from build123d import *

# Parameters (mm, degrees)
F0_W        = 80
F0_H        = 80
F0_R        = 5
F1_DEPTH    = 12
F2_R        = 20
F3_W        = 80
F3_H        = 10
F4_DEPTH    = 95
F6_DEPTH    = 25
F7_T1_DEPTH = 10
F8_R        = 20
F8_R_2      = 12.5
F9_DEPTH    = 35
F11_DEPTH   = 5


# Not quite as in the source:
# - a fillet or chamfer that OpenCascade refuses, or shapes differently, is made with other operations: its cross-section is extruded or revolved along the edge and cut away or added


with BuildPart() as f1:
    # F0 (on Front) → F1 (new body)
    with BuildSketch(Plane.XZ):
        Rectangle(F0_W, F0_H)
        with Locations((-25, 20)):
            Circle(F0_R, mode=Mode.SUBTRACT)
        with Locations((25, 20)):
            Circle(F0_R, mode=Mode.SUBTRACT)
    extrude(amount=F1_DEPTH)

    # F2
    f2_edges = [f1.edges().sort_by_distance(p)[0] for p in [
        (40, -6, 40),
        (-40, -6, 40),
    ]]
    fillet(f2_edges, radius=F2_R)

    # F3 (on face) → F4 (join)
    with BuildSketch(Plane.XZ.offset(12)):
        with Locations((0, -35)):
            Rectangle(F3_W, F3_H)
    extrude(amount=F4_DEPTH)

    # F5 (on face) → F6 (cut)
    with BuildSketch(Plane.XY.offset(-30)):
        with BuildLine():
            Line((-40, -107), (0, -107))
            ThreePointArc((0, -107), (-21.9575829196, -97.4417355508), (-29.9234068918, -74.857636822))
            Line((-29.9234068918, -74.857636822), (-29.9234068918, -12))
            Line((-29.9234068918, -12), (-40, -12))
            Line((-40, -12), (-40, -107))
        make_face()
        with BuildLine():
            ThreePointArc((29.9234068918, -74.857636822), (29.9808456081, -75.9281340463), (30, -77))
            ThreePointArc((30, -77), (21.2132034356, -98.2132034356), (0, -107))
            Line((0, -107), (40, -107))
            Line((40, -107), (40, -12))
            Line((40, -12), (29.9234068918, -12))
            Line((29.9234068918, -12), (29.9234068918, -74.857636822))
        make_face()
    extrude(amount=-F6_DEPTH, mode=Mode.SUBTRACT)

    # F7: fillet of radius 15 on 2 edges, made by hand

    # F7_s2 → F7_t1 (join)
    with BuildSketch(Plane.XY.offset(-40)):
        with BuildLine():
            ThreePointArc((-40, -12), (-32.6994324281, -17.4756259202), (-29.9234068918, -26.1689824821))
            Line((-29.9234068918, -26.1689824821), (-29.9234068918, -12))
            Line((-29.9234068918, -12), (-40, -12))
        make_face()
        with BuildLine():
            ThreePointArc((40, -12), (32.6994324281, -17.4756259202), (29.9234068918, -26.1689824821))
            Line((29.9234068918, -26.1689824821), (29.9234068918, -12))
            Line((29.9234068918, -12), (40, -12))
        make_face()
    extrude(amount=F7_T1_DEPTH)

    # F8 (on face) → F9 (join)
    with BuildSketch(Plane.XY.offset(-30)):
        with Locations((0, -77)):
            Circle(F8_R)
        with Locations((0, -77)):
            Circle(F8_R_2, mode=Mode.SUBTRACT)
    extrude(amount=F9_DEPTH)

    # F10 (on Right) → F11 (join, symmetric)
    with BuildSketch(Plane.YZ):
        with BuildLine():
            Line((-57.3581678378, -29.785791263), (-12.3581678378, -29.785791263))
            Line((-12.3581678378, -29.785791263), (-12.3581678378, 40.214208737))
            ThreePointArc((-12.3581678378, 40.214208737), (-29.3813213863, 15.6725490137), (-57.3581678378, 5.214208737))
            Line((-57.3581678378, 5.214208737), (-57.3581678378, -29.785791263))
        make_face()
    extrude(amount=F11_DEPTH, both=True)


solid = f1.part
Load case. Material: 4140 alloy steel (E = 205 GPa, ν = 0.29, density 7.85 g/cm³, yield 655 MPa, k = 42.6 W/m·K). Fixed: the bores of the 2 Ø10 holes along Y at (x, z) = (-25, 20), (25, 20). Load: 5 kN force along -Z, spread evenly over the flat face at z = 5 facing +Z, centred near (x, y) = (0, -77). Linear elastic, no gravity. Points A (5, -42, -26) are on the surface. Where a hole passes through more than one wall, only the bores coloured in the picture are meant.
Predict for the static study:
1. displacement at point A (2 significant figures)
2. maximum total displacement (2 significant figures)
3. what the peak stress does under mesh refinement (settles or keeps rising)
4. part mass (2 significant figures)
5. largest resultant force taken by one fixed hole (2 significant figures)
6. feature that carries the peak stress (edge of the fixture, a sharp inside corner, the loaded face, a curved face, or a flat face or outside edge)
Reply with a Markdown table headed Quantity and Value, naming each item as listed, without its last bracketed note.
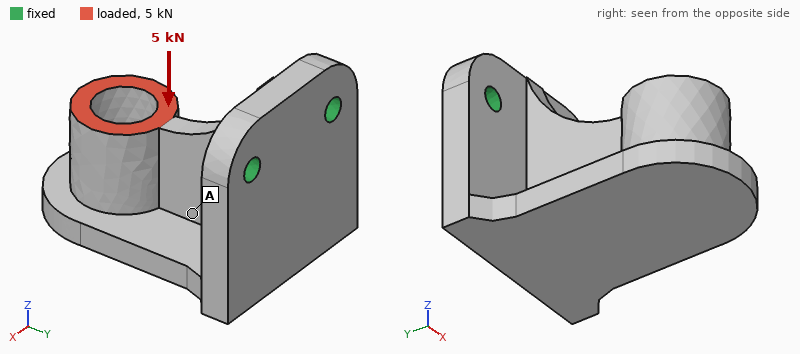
| Quantity | Value |
|---|---|
| displacement at point A | 0.41 mm |
| maximum total displacement | 1.6 mm |
| what the peak stress does under mesh refinement | keeps rising |
| part mass | 1.4 kg |
| largest resultant force taken by one fixed hole | 2.6 kN |
| feature that carries the peak stress | edge of the fixture |
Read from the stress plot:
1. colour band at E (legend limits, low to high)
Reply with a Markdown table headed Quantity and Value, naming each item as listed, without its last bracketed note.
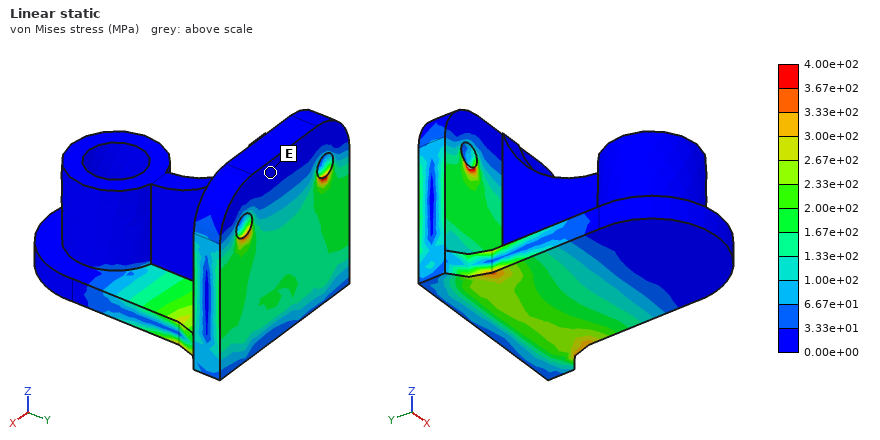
| Quantity | Value |
|---|---|
| colour band at E | 0.00e+00 to 3.33e+01 MPa |
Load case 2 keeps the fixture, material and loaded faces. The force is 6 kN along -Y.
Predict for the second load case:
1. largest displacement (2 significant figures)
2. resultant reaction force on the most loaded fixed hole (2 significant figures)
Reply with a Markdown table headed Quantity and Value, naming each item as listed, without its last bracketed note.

| Quantity | Value |
|---|---|
| largest displacement | 1.1 mm |
| resultant reaction force on the most loaded fixed hole | 3.0 kN |
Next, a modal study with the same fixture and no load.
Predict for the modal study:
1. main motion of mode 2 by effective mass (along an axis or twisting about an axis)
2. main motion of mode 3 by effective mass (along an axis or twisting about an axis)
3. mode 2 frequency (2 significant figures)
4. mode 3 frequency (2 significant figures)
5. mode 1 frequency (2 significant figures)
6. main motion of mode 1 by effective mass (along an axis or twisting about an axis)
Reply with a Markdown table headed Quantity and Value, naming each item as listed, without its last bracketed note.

| Quantity | Value |
|---|---|
| main motion of mode 2 by effective mass | along X |
| main motion of mode 3 by effective mass | along Y |
| mode 2 frequency | 840 Hz |
| mode 3 frequency | 1100 Hz |
| mode 1 frequency | 470 Hz |
| main motion of mode 1 by effective mass | along Z |
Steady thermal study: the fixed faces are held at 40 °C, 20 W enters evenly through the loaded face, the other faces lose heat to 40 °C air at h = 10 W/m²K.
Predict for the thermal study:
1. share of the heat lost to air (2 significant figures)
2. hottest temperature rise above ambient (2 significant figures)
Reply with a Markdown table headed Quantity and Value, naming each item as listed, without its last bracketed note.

| Quantity | Value |
|---|---|
| share of the heat lost to air | 52 % |
| hottest temperature rise above ambient | 59 K |
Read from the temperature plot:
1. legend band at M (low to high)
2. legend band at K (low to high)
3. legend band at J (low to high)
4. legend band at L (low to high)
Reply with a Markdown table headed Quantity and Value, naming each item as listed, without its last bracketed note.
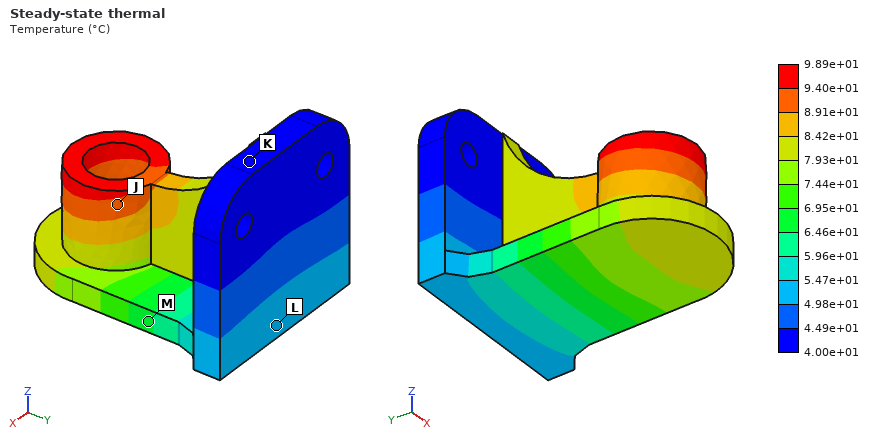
| Quantity | Value |
|---|---|
| legend band at M | 6.46e+01 to 6.95e+01 °C |
| legend band at K | 4.00e+01 to 4.49e+01 °C |
| legend band at J | 8.91e+01 to 9.40e+01 °C |
| legend band at L | 4.98e+01 to 5.47e+01 °C |
